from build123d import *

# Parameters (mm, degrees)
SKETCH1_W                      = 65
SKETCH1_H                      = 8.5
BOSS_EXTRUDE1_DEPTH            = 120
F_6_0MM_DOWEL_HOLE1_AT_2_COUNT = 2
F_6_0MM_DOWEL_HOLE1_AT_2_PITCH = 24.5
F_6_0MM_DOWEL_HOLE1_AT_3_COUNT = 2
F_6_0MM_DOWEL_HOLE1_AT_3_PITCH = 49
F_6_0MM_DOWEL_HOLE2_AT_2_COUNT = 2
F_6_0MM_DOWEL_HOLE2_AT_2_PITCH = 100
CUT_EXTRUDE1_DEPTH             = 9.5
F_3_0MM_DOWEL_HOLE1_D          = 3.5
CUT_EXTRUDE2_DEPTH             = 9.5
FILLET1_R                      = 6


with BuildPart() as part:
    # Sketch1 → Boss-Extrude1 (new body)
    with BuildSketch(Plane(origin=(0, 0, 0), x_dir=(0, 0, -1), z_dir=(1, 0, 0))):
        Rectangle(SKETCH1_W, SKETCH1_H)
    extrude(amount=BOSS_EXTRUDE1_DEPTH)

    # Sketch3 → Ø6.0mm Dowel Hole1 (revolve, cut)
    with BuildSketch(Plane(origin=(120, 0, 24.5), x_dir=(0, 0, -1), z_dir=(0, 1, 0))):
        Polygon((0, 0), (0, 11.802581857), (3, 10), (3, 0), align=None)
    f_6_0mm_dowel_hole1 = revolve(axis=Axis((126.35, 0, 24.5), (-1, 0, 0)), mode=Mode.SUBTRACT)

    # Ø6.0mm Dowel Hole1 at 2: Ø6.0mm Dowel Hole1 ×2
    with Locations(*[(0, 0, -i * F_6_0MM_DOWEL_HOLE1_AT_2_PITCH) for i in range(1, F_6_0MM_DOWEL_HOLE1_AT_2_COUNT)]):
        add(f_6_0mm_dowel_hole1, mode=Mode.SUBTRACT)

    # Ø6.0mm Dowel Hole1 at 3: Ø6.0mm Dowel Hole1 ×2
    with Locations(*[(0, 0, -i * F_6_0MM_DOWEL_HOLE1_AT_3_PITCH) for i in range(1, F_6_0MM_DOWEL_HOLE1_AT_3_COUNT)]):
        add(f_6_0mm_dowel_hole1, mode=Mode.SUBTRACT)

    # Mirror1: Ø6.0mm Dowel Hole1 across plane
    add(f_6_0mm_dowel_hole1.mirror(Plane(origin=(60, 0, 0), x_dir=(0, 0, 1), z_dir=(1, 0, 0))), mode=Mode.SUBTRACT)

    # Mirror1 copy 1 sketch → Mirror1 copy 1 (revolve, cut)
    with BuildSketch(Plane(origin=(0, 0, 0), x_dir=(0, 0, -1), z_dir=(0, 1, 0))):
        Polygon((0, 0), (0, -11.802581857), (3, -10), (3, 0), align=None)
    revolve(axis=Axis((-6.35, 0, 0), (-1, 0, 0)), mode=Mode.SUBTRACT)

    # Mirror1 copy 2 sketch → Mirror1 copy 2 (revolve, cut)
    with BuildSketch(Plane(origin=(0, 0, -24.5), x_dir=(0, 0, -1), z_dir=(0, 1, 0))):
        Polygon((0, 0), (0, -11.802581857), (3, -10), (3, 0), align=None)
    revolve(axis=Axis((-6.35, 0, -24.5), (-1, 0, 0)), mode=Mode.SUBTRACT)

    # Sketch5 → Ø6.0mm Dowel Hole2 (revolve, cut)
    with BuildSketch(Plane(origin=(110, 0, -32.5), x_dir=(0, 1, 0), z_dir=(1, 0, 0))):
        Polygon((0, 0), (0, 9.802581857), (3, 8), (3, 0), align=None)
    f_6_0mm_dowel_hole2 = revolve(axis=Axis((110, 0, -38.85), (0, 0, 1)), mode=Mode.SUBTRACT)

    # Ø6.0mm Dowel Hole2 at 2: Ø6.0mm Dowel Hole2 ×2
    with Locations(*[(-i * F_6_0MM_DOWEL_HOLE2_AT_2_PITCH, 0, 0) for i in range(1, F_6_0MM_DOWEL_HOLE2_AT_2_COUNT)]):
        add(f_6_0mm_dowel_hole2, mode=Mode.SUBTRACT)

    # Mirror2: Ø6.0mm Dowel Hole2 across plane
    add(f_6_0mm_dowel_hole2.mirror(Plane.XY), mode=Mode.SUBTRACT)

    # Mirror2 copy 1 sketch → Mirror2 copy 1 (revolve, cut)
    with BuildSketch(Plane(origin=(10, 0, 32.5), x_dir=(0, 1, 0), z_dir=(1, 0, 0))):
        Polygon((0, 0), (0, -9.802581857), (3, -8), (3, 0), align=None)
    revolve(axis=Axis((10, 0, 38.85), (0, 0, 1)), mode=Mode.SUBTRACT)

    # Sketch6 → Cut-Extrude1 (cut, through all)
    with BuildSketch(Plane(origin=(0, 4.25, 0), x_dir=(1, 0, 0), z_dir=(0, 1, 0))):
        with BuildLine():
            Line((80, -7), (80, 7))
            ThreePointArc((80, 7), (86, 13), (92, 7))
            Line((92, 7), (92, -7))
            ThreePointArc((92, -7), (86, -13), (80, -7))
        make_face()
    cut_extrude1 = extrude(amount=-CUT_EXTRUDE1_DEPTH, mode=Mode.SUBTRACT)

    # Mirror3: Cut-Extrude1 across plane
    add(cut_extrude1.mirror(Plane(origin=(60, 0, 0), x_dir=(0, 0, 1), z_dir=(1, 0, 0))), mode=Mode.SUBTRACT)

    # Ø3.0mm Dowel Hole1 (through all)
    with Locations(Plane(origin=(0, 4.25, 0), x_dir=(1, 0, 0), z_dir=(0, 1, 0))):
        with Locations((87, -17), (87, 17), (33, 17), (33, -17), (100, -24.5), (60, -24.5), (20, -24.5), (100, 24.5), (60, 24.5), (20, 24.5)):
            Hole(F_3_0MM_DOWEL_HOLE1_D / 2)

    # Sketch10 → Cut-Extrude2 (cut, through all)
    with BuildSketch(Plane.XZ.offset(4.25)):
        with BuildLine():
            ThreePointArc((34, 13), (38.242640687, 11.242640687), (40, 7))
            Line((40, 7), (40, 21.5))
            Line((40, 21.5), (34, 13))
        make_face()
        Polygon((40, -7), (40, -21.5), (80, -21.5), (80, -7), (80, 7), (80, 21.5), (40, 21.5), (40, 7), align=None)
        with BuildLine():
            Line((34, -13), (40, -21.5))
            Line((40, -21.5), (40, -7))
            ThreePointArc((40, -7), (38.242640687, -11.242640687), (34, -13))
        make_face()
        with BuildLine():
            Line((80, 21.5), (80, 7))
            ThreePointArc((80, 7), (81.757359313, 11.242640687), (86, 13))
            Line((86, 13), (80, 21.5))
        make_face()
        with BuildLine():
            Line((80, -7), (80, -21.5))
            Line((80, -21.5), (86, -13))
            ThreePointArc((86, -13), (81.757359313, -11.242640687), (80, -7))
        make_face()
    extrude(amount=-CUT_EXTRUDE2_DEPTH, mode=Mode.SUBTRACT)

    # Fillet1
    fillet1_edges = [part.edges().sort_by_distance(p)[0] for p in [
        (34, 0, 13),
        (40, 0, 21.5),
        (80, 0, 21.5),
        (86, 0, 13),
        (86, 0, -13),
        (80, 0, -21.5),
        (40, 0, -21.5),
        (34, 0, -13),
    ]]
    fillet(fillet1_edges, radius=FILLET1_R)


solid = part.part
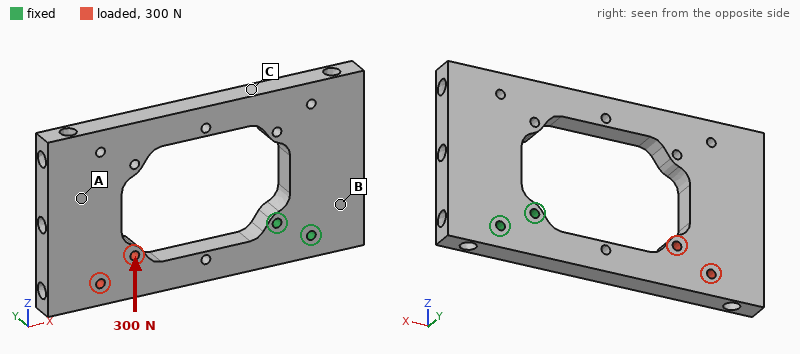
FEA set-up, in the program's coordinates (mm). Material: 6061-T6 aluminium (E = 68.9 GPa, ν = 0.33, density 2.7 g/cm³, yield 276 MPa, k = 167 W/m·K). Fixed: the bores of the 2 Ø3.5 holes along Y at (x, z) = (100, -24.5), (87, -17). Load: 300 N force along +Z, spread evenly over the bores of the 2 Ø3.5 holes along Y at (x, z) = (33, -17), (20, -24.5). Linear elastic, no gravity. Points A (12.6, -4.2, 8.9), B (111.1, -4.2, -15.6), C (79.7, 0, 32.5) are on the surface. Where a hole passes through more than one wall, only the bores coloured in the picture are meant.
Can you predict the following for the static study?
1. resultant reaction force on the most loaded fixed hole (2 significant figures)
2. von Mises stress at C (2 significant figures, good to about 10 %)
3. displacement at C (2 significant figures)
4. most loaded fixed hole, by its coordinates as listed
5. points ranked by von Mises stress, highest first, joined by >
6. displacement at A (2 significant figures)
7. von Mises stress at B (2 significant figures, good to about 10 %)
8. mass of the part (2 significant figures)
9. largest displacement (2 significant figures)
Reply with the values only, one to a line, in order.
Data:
1.4 kN
10 MPa
31 µm
(87, -17)
C > B > A
72 µm
5.8 MPa
110 g
81 µm
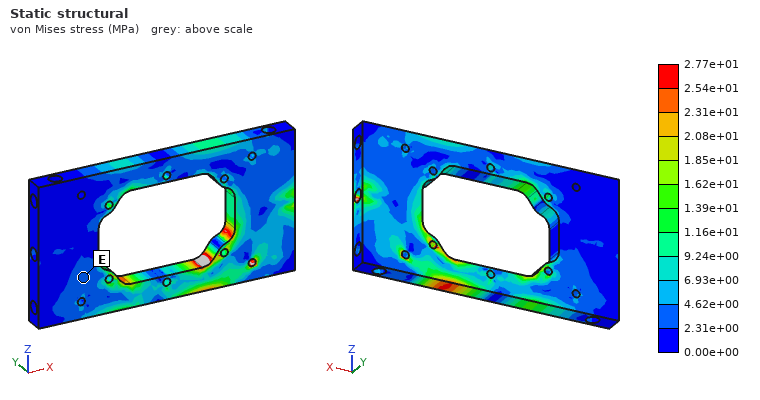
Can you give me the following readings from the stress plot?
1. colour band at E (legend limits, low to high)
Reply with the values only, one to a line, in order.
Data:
2.31e+00 to 4.62e+00 MPa
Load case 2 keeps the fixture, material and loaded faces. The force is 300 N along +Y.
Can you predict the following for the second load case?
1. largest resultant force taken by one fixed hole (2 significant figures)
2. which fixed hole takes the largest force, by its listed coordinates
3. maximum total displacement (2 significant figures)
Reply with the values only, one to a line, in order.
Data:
990 N
(87, -17)
0.70 mm
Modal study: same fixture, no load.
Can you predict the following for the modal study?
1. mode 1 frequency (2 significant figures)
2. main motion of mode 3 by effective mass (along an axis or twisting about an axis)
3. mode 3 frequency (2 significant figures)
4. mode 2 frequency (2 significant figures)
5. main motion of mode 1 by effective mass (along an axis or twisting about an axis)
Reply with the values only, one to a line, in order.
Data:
460 Hz
along Z
1300 Hz
1300 Hz
along Y
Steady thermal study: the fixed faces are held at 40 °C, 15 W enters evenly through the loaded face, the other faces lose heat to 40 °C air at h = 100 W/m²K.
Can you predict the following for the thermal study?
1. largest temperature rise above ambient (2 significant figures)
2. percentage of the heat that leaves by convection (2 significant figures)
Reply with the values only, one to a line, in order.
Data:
17 K
70 %
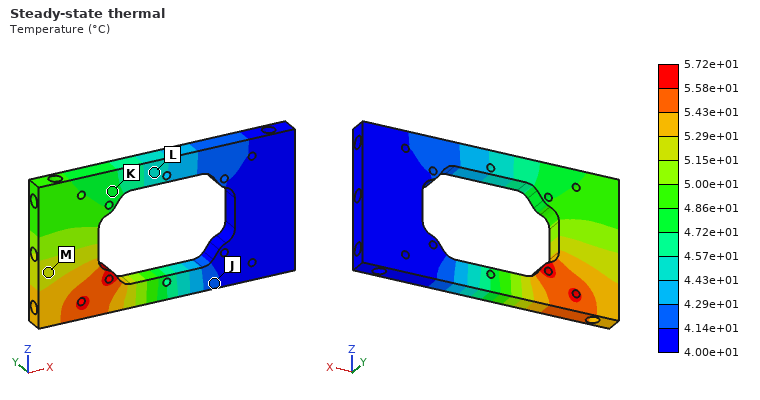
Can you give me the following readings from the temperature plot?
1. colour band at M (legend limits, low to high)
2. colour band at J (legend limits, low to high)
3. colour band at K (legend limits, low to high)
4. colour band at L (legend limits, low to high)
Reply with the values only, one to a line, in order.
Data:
5.15e+01 to 5.29e+01 °C
4.14e+01 to 4.29e+01 °C
4.72e+01 to 4.86e+01 °C
4.43e+01 to 4.57e+01 °C
